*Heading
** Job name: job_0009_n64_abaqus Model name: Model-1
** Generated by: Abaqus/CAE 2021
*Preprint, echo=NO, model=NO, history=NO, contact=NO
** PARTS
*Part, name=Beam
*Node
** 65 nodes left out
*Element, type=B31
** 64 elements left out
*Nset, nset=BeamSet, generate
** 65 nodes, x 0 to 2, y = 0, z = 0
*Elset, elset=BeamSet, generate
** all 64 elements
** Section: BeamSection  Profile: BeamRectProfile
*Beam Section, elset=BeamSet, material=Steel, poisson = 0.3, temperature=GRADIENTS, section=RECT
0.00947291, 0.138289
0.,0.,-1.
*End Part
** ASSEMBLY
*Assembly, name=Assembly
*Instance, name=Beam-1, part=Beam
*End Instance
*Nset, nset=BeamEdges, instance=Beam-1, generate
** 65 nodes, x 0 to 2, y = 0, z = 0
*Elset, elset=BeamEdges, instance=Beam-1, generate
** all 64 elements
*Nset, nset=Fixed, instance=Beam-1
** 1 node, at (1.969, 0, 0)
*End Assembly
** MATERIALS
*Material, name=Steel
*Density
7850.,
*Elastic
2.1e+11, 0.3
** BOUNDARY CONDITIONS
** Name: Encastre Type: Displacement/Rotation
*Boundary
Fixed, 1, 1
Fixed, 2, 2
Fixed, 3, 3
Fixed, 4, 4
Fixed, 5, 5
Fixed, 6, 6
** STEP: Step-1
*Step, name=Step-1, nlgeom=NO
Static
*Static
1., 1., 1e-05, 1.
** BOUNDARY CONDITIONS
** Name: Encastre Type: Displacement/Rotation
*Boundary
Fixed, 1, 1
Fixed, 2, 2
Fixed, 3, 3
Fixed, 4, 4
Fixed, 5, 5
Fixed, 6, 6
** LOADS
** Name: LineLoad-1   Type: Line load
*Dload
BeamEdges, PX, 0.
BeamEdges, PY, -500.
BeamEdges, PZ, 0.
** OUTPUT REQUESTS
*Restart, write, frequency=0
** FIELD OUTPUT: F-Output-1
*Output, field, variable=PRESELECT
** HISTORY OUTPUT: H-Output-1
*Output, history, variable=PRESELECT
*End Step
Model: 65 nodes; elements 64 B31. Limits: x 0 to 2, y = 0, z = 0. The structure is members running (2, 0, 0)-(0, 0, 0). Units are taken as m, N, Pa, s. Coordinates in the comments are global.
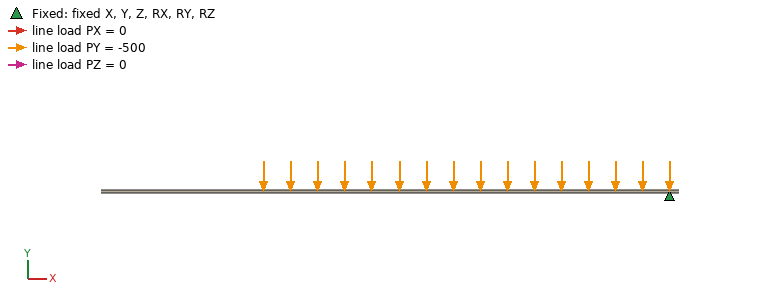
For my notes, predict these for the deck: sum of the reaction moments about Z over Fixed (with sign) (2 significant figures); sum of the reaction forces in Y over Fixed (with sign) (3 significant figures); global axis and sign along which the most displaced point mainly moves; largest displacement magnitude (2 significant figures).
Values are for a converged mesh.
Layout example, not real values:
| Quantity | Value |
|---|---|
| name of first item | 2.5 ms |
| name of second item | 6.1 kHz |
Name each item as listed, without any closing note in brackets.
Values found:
| Quantity | Value |
|---|---|
| sum of the reaction moments about Z over Fixed (with sign) | -970 N·m |
| sum of the reaction forces in Y over Fixed (with sign) | 1000 N |
| global axis and sign along which the most displaced point mainly moves | -Y |
| largest displacement magnitude | 0.0022 m |
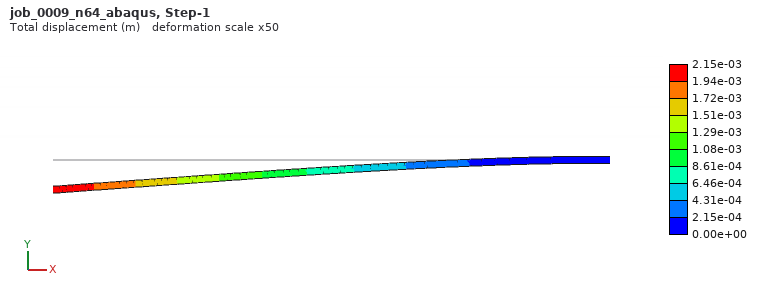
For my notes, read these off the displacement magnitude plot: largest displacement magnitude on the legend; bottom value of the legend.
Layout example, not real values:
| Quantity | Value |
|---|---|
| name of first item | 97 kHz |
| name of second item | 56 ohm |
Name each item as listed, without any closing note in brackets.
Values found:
| Quantity | Value |
|---|---|
| largest displacement magnitude on the legend | 2.15e-03 m |
| bottom value of the legend | 0.00e+00 m |
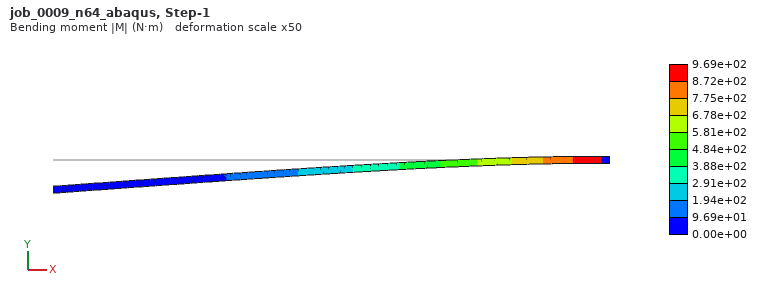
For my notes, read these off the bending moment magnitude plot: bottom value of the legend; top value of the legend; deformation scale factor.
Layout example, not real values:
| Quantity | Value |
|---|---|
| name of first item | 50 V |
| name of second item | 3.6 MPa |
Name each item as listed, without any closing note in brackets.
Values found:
| Quantity | Value |
|---|---|
| bottom value of the legend | 0.00e+00 N·m |
| top value of the legend | 9.69e+02 N·m |
| deformation scale factor | 50 |
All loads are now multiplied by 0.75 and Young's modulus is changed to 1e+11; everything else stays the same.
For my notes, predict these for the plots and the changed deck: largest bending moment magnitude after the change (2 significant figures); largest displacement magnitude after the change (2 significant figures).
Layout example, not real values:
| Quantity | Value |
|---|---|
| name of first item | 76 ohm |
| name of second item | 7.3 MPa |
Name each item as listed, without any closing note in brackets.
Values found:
| Quantity | Value |
|---|---|
| largest bending moment magnitude after the change | 730 N·m |
| largest displacement magnitude after the change | 0.0034 m |
